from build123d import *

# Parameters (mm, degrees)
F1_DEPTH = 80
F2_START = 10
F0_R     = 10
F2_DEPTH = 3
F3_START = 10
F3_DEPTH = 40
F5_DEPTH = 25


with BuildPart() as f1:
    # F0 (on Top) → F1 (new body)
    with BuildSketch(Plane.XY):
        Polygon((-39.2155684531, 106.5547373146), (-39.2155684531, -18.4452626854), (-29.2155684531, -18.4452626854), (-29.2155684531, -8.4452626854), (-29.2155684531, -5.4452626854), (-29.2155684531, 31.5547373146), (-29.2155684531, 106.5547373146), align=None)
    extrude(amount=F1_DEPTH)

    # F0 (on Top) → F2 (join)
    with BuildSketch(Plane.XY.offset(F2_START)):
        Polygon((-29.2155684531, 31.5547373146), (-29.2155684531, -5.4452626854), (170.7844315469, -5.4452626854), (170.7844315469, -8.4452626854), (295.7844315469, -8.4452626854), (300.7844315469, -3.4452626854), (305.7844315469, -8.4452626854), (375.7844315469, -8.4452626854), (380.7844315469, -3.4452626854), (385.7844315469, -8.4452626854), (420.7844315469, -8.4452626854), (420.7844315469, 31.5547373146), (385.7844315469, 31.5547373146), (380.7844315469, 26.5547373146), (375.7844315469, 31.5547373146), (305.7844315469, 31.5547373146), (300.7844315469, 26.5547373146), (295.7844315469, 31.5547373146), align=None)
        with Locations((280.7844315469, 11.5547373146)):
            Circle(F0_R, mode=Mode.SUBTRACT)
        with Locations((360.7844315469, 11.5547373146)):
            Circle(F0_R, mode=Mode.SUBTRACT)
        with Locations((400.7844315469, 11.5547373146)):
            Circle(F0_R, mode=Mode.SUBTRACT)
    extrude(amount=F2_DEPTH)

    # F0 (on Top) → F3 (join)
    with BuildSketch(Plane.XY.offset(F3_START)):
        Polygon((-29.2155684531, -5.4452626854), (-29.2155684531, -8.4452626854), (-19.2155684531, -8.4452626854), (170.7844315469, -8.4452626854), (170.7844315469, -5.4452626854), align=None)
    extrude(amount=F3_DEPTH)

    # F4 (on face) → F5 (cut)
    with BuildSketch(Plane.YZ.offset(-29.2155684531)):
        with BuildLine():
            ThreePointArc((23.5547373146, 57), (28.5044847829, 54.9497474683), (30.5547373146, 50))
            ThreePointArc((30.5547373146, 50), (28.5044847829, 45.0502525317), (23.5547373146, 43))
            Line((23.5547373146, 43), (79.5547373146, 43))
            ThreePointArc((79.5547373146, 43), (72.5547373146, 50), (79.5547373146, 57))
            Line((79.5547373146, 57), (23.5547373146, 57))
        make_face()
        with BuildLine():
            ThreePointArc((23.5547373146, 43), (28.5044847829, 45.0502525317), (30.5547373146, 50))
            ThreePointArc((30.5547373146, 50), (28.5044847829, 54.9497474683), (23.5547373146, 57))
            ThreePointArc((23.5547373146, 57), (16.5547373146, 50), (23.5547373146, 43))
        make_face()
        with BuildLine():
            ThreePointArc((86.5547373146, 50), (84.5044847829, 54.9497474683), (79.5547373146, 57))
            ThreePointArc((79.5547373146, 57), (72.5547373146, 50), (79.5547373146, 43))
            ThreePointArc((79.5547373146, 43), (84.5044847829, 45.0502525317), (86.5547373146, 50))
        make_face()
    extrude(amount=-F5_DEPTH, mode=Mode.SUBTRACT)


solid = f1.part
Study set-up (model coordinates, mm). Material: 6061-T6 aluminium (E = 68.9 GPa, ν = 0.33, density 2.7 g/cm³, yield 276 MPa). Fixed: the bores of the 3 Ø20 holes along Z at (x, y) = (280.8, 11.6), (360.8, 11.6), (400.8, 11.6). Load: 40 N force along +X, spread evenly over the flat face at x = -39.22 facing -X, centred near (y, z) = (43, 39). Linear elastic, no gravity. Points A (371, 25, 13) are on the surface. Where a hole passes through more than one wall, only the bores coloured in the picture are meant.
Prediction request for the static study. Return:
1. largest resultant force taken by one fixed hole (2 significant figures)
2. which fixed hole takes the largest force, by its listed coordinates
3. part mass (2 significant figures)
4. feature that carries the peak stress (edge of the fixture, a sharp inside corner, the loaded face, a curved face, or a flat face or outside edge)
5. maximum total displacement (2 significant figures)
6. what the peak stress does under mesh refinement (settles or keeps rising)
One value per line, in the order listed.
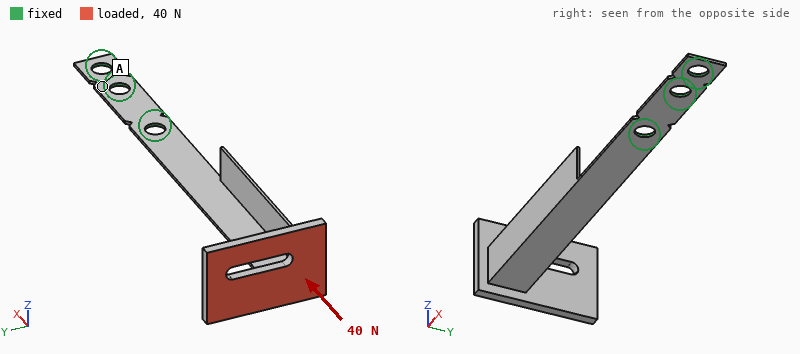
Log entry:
39 N
(280.8, 11.6)
440 g
a sharp inside corner
5.3 mm
keeps rising
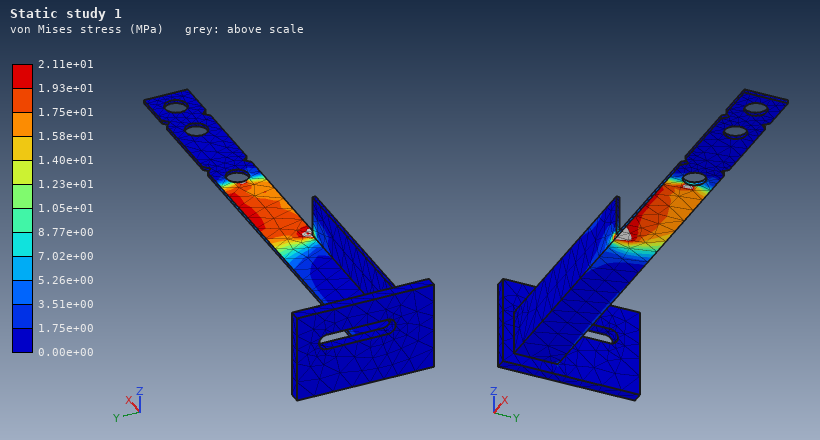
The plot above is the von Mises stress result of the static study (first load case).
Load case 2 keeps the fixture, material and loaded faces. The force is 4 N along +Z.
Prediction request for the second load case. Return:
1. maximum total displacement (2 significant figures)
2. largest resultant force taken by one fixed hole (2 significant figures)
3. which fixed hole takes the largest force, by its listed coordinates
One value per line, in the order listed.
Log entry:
5.1 mm
3.9 N
(280.8, 11.6)
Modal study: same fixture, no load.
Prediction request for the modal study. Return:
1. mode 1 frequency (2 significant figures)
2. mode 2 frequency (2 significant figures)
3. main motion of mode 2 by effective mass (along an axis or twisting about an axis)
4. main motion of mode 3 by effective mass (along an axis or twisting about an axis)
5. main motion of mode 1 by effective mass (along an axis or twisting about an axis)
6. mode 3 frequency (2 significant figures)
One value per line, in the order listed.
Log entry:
8.6 Hz
38 Hz
along Y
along Y
along Z
110 Hz
